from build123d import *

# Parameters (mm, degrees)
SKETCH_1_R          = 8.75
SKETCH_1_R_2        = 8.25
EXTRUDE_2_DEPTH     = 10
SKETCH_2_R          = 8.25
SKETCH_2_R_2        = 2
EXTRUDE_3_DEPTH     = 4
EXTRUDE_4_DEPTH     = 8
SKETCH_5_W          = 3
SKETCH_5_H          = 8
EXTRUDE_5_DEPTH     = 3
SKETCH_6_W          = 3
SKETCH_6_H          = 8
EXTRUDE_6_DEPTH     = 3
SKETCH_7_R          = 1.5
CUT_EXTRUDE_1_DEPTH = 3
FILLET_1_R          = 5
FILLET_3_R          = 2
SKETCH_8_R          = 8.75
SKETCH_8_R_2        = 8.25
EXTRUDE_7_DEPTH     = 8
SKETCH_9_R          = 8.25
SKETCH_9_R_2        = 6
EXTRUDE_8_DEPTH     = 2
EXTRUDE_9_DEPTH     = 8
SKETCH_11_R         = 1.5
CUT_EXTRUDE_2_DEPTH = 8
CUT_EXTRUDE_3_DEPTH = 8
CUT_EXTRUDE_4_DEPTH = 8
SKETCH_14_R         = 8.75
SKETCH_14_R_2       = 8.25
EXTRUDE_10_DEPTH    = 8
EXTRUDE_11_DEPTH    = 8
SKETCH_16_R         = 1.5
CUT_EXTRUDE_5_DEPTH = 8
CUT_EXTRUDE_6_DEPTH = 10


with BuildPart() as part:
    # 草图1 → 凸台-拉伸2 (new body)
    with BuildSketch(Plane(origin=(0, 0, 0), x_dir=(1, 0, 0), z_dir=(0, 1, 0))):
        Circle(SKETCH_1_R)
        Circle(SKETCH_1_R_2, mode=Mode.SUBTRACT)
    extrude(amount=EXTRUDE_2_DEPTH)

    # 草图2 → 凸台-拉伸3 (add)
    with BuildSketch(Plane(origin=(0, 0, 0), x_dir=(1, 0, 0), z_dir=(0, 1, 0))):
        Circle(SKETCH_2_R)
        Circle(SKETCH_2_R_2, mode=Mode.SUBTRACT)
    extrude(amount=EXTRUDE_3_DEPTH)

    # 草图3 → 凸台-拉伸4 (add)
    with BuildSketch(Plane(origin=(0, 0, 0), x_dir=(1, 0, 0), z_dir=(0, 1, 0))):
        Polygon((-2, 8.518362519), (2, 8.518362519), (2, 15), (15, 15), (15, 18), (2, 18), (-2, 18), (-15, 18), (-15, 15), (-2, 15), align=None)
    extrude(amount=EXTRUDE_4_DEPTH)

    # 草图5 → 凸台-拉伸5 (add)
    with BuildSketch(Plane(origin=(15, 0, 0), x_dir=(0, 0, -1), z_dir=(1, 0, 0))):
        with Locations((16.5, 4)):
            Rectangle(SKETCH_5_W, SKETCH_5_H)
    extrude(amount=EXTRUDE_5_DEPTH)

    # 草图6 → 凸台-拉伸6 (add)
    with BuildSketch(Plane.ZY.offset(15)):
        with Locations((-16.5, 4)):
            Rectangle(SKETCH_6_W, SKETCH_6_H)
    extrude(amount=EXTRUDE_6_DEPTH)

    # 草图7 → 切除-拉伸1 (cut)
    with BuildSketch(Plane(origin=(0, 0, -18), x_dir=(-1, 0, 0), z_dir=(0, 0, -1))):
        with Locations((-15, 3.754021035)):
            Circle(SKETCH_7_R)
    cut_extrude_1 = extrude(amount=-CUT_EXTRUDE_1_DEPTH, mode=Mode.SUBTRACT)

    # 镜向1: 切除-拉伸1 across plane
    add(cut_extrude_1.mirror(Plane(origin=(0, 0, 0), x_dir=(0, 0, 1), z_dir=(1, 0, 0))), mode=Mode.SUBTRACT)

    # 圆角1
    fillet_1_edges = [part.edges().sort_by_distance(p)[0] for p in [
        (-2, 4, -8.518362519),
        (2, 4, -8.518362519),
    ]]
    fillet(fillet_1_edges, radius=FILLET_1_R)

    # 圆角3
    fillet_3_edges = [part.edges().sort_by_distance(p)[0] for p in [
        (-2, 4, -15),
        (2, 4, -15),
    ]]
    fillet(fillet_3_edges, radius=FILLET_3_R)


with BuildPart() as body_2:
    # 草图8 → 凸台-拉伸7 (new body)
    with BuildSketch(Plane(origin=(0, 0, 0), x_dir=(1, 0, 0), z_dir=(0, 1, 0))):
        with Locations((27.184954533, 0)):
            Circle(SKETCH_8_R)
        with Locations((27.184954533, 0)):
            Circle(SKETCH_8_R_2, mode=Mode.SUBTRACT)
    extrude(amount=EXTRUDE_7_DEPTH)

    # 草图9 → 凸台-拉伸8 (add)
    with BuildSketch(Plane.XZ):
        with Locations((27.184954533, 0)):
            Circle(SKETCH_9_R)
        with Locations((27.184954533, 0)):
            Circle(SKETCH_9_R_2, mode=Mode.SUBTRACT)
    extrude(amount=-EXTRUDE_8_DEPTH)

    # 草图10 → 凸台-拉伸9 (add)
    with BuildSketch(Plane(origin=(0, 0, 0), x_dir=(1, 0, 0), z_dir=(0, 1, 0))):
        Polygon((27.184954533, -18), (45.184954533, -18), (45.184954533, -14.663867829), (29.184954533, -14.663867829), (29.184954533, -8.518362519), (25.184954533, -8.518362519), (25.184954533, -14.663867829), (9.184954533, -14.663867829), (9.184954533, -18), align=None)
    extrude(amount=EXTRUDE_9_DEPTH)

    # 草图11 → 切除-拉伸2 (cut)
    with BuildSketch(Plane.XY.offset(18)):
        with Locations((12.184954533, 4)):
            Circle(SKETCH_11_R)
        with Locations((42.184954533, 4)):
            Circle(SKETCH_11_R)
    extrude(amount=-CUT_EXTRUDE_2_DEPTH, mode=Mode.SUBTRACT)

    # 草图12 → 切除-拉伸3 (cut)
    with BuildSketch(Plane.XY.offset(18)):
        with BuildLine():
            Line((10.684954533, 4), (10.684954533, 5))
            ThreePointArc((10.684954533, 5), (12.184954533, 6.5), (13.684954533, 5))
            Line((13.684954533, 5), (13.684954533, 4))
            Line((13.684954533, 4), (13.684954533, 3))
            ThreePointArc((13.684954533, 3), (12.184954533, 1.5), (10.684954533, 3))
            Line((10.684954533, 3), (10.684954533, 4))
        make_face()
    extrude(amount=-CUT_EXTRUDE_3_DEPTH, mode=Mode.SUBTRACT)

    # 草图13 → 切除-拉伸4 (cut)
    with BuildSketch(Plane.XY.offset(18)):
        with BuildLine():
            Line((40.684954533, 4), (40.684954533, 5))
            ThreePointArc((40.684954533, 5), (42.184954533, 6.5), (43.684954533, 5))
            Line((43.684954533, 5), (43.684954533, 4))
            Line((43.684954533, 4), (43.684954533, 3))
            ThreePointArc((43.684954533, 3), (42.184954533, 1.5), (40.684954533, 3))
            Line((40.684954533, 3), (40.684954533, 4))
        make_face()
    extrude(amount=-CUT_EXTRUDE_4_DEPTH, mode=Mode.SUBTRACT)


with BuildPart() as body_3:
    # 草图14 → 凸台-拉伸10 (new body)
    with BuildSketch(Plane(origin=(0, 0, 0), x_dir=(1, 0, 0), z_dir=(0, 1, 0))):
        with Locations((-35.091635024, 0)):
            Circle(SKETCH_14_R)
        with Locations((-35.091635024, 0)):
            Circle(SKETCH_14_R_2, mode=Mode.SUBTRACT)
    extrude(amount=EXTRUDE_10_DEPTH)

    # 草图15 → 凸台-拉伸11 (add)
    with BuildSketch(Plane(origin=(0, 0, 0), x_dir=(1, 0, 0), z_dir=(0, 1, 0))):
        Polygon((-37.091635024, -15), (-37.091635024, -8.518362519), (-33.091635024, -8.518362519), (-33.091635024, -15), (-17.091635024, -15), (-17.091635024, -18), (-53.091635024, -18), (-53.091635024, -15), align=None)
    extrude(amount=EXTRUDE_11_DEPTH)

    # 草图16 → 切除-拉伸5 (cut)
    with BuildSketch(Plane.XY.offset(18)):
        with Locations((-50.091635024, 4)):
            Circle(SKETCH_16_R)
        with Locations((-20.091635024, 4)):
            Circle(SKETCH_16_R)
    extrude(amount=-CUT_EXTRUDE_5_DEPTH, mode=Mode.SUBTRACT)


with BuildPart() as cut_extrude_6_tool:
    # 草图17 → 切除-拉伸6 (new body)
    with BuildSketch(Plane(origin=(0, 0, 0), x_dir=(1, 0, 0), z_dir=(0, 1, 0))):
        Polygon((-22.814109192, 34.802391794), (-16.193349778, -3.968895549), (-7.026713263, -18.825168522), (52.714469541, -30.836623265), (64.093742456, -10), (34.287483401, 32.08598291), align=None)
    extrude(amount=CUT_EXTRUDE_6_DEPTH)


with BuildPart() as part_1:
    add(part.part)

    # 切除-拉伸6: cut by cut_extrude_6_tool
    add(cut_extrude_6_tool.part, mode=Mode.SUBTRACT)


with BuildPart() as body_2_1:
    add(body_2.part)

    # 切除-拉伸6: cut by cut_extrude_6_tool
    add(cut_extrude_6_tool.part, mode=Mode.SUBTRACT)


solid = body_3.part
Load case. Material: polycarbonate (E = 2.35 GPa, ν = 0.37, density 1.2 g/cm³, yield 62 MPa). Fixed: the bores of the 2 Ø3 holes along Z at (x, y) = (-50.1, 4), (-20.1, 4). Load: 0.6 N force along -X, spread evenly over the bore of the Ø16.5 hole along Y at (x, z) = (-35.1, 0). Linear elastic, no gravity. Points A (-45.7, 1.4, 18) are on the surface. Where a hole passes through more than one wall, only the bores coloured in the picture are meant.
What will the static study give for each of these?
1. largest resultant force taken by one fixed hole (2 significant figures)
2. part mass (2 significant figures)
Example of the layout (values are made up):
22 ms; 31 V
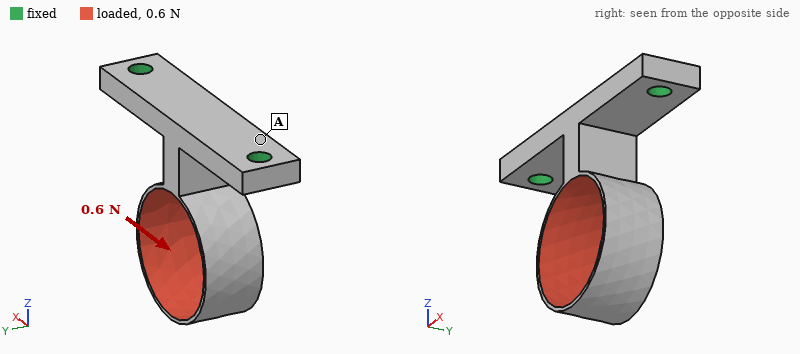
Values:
0.59 N; 1.5 g
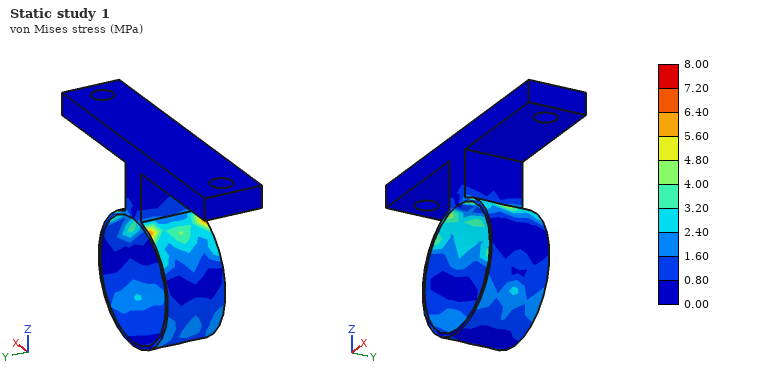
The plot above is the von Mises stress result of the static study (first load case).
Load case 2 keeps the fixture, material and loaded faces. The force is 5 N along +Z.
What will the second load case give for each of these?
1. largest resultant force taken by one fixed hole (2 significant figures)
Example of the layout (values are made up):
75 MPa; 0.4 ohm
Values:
2.6 N
